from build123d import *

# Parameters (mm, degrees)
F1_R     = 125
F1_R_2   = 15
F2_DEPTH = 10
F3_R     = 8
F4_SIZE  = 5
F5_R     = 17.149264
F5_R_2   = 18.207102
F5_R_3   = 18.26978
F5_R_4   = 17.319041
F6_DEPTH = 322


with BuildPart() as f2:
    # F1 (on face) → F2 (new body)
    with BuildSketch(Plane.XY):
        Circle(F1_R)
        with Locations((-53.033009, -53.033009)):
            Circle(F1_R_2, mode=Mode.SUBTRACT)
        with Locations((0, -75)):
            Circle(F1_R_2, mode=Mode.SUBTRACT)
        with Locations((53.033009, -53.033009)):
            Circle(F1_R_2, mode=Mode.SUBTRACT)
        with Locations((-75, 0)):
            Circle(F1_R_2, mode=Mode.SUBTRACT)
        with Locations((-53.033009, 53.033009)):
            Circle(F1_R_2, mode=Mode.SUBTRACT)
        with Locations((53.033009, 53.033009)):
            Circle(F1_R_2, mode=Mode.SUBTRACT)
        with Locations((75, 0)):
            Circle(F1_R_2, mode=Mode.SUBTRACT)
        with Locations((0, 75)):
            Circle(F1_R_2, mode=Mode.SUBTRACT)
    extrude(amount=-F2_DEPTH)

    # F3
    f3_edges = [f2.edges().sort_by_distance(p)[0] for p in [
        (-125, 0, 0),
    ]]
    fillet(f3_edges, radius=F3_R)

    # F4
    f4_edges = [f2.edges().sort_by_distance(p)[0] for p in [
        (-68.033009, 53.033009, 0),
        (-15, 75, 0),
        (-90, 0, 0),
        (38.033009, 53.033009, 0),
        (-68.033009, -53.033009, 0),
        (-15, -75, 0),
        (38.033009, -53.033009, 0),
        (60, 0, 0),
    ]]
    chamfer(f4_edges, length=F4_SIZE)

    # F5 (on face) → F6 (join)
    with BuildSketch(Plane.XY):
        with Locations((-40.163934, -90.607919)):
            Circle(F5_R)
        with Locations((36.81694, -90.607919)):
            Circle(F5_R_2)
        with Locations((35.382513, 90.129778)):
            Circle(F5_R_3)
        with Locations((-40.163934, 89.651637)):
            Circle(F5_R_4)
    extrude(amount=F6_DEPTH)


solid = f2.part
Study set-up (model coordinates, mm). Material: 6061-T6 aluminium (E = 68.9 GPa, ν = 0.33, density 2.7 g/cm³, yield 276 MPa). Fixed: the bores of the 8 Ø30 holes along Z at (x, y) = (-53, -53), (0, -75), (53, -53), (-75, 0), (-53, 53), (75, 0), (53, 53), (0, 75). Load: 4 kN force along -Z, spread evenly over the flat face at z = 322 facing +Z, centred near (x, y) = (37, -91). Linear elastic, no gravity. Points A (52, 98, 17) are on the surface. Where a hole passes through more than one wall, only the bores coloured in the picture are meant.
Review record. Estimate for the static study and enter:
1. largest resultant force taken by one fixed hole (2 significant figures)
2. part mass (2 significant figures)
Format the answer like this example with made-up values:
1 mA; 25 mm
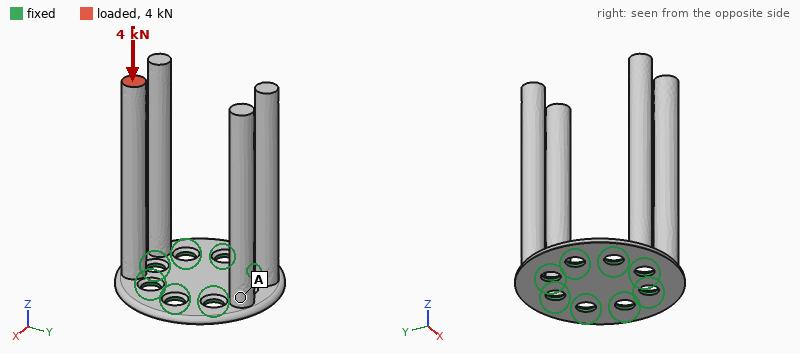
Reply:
2.3 kN; 4.6 kg
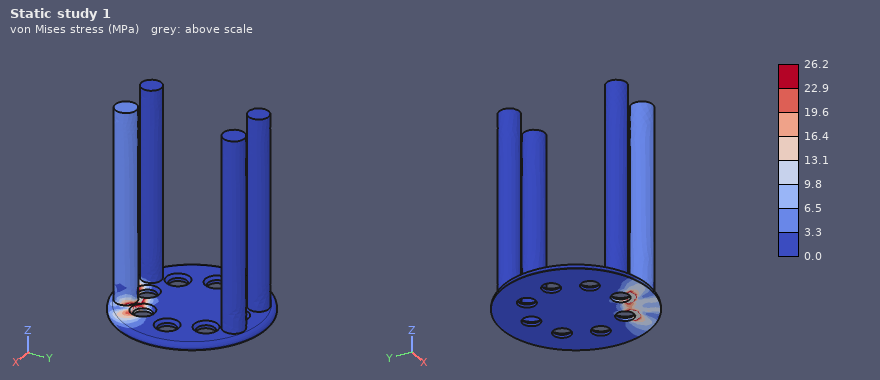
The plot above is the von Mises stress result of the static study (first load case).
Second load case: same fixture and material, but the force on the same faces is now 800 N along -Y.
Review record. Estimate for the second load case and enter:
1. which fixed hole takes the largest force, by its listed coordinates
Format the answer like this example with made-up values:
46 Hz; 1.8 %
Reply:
(0, -75)
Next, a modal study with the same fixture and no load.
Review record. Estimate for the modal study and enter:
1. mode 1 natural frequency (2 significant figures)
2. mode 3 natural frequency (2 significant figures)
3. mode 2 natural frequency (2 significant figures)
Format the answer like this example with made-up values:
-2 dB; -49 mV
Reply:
140 Hz; 150 Hz; 140 Hz
